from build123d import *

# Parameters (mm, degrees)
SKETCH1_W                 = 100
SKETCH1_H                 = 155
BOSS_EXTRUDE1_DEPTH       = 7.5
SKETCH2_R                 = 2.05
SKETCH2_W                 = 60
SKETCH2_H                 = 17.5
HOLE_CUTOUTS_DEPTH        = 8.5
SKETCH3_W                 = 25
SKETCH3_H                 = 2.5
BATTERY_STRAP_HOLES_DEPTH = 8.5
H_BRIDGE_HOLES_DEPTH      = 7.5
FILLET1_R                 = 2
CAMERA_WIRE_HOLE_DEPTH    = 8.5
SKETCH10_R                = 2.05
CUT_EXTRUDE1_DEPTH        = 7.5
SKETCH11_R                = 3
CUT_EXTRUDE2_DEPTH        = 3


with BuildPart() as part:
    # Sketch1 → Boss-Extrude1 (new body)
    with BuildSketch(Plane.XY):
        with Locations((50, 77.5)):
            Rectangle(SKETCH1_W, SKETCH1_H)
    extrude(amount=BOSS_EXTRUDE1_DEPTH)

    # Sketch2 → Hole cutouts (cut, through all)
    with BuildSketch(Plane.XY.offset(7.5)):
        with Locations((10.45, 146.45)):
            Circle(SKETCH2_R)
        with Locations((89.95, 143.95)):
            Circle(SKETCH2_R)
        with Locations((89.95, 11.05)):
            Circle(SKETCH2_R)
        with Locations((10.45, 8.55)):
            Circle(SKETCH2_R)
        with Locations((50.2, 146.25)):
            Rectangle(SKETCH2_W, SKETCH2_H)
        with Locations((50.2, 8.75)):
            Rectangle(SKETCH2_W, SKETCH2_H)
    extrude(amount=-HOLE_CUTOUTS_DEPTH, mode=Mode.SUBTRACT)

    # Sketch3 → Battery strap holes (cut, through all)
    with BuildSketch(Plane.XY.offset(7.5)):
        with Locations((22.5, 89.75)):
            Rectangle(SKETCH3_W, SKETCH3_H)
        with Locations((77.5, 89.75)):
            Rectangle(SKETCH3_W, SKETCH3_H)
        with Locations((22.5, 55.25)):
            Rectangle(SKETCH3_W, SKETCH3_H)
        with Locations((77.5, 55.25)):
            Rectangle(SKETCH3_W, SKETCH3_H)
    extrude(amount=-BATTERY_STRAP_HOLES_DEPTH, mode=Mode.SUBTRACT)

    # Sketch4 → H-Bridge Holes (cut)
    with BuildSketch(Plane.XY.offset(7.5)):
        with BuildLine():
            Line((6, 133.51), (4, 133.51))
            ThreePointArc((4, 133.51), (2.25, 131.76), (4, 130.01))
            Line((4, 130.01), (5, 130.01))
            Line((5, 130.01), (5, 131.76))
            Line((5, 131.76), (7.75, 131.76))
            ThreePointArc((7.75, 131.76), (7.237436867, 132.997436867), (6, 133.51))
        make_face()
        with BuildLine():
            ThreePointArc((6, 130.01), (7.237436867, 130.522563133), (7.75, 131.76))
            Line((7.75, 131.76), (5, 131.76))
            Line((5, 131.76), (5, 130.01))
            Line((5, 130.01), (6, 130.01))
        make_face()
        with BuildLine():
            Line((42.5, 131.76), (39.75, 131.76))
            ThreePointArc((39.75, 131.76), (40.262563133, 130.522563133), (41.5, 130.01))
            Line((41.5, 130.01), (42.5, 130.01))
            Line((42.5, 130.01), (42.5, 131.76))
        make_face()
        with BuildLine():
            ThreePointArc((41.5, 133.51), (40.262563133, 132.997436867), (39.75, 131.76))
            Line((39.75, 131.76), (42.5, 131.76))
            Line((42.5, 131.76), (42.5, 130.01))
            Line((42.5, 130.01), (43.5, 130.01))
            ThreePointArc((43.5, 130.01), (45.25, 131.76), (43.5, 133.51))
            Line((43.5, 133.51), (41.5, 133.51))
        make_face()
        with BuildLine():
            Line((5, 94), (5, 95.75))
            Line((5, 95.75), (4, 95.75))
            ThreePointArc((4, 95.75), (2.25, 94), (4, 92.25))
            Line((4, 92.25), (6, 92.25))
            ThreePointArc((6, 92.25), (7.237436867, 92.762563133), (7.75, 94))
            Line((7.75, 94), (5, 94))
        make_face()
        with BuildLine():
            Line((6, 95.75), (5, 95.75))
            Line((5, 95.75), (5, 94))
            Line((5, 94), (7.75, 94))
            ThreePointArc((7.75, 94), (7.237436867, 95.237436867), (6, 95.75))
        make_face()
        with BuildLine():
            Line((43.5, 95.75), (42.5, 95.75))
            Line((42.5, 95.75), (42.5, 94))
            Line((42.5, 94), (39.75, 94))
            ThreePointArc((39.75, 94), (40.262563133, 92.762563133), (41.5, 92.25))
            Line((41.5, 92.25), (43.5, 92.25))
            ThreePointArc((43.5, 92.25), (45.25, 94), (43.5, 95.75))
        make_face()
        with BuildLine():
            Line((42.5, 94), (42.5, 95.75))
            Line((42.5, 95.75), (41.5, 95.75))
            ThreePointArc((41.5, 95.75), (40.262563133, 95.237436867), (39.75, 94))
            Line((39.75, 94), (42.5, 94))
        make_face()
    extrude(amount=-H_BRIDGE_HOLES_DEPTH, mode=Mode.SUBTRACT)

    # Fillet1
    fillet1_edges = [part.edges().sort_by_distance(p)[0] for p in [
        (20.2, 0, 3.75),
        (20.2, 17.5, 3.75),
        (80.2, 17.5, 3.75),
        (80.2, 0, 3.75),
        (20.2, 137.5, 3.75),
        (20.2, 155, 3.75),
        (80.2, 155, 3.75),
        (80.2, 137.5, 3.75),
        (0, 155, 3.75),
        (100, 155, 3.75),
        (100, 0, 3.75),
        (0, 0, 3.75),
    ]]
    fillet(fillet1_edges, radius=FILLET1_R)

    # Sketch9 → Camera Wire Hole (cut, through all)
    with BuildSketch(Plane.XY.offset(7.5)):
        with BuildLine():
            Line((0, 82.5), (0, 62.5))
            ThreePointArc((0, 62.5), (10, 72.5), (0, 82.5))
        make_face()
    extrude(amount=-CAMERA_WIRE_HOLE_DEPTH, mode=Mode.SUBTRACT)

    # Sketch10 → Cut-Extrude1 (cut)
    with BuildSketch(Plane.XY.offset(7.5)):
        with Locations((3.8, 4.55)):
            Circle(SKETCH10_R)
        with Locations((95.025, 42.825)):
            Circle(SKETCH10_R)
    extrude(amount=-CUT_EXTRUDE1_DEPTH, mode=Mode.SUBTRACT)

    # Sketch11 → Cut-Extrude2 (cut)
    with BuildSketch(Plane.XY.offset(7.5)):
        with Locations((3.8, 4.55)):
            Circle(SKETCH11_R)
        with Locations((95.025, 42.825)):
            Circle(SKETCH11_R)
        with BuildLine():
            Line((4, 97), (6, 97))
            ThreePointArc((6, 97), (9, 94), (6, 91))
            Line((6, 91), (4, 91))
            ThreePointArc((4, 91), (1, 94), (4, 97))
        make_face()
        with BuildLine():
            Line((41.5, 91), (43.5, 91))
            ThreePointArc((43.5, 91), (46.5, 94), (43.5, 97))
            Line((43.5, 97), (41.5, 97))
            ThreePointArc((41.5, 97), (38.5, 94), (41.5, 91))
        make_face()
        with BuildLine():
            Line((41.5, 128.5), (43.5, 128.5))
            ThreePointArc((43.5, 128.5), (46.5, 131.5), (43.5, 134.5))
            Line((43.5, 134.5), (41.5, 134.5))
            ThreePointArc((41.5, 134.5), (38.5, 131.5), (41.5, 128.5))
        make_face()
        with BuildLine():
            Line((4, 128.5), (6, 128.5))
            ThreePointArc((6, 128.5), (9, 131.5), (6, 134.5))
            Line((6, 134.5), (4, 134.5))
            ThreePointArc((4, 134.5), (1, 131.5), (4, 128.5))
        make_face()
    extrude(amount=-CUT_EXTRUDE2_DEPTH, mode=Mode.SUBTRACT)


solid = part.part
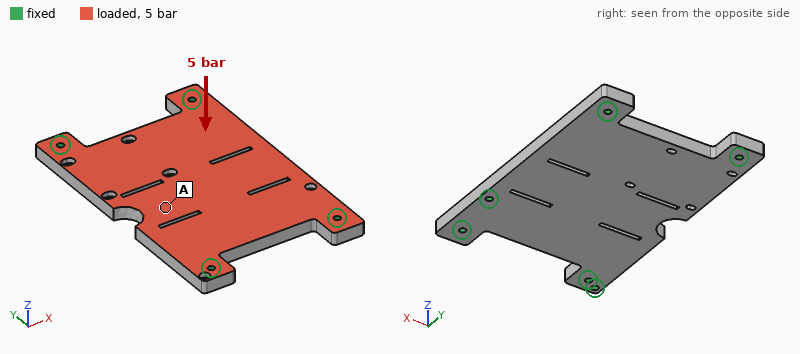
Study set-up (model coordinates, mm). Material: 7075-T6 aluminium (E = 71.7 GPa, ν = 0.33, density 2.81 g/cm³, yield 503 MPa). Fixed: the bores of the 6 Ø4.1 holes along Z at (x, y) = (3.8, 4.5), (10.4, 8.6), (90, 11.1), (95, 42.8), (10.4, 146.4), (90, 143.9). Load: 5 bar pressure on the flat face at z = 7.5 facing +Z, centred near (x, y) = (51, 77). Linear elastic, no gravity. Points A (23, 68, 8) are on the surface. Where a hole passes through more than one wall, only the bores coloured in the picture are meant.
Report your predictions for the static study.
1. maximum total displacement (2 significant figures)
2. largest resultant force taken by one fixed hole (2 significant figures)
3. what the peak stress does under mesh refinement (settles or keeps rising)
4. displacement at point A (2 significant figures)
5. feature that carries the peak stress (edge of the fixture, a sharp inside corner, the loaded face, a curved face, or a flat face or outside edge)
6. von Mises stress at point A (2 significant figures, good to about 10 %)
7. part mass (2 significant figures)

0.35 mm
2.2 kN
keeps rising
0.29 mm
edge of the fixture
27 MPa
270 g
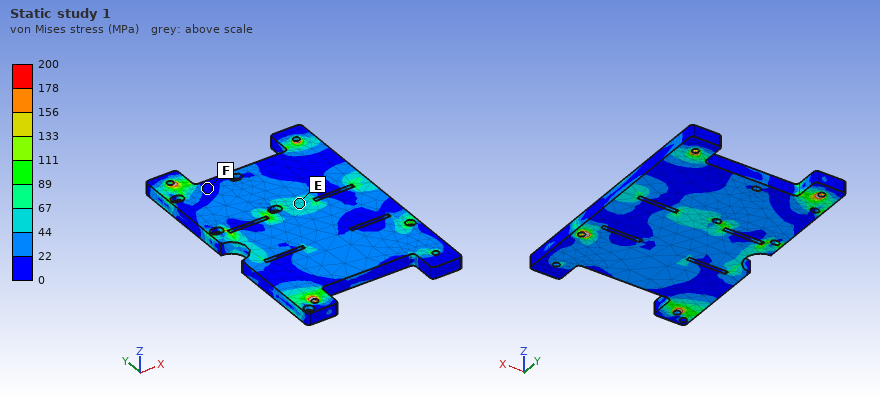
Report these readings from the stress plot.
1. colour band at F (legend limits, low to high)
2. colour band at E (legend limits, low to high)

0 to 22 MPa
44 to 67 MPa
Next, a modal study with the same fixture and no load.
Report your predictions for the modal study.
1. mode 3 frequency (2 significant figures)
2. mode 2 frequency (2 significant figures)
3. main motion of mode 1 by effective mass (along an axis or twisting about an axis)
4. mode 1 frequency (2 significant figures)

4100 Hz
3200 Hz
along Z
1700 Hz
